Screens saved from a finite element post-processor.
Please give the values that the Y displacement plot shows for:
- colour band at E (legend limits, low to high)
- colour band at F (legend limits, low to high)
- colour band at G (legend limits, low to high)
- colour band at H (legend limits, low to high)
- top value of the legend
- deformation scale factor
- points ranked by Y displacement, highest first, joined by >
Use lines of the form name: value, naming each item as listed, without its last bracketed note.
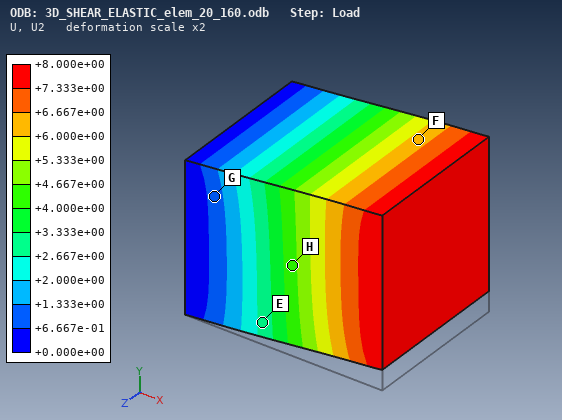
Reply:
colour band at E: +2.667e+00 to +3.333e+00
colour band at F: +6.000e+00 to +6.667e+00
colour band at G: +6.667e-01 to +1.333e+00
colour band at H: +4.000e+00 to +4.667e+00
top value of the legend: +8.000e+00
deformation scale factor: 2
points ranked by Y displacement, highest first, joined by >: F > H > E > G
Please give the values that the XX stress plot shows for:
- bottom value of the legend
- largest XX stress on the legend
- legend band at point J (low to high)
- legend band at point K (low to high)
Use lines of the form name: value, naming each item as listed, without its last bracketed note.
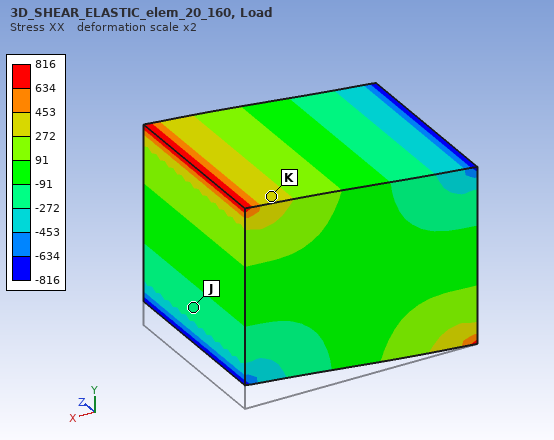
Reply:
bottom value of the legend: -816
largest XX stress on the legend: 816
legend band at point J: -272 to -91
legend band at point K: 272 to 453
